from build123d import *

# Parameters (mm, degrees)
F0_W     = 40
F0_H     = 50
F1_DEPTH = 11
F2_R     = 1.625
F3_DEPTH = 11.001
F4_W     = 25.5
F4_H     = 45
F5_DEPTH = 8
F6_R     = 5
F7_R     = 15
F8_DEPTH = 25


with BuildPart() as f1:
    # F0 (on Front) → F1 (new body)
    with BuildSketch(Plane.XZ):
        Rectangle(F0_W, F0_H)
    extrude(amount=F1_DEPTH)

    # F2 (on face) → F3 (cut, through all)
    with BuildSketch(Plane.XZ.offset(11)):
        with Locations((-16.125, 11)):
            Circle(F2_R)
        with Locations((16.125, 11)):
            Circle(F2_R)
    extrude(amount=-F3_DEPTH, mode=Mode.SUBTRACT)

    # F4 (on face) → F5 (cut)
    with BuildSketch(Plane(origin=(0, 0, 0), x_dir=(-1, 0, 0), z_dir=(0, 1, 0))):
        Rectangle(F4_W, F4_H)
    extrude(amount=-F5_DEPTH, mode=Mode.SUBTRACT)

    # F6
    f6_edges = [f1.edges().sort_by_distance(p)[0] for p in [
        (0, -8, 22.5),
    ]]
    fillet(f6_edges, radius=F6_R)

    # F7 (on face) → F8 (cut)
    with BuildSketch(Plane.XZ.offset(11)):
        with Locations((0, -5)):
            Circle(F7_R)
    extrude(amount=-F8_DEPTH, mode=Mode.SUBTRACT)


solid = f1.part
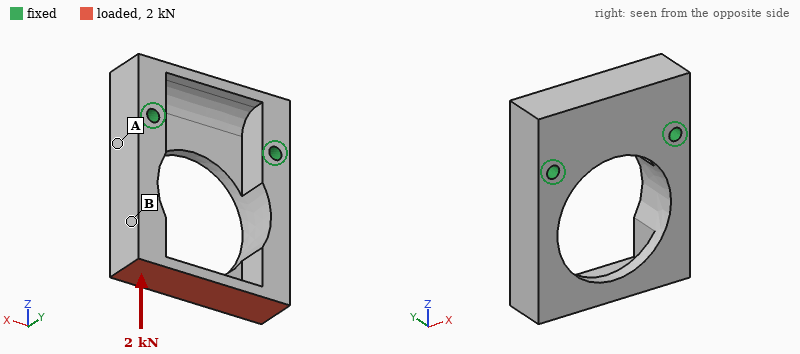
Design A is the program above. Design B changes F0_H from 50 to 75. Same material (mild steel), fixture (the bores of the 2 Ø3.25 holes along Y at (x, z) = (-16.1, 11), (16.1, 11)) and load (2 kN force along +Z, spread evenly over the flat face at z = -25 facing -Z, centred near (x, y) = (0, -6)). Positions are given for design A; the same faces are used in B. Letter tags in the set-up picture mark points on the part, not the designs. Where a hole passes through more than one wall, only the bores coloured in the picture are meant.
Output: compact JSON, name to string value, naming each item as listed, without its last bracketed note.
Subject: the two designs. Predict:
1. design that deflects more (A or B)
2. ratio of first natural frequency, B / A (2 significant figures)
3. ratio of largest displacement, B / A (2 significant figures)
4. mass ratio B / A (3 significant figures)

{"design that deflects more": "A", "ratio of first natural frequency, B / A": "0.45", "ratio of largest displacement, B / A": "0.17", "mass ratio B / A": "2.07"}
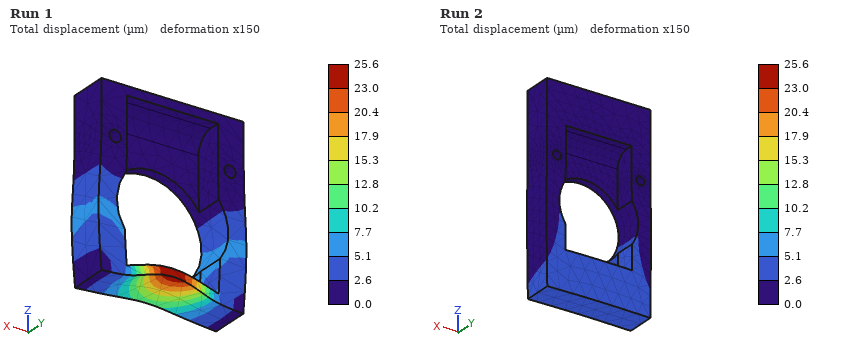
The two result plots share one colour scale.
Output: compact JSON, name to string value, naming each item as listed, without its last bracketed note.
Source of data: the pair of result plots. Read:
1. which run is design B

{"which run is design B": "Run 2"}
